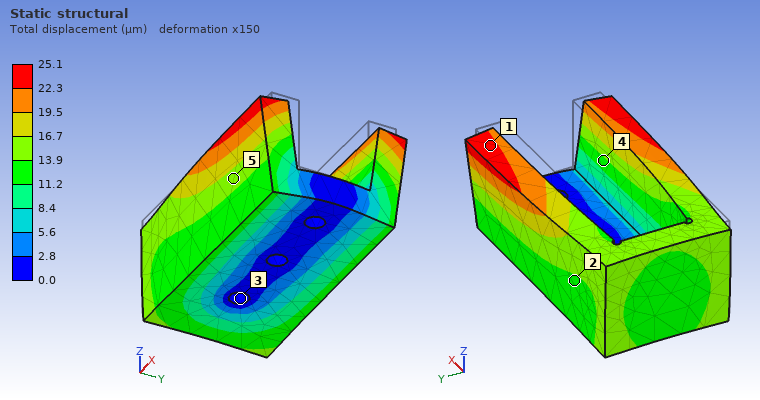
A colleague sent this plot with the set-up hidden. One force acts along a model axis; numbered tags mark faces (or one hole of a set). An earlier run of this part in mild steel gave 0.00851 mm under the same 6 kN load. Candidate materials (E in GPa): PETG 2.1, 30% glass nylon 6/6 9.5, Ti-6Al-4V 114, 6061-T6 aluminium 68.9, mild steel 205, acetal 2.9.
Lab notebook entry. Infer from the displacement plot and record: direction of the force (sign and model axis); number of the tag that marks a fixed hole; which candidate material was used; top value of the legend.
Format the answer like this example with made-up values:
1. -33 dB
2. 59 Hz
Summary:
1. -Z
2. 3
3. 6061-T6 aluminium
4. 25.1 µm
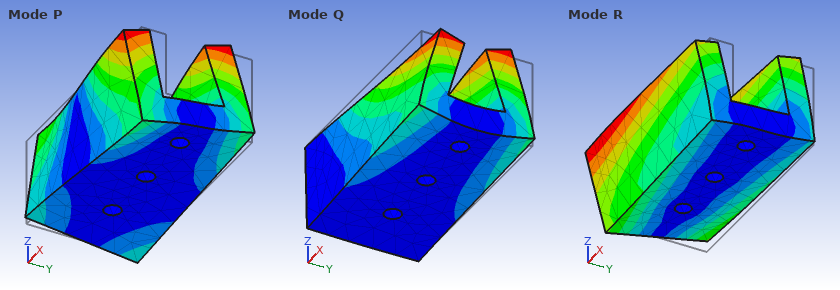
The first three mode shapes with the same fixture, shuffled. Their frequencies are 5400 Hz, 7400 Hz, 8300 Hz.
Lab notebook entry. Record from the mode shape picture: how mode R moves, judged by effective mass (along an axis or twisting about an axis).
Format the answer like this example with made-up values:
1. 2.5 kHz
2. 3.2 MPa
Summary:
1. along Y
